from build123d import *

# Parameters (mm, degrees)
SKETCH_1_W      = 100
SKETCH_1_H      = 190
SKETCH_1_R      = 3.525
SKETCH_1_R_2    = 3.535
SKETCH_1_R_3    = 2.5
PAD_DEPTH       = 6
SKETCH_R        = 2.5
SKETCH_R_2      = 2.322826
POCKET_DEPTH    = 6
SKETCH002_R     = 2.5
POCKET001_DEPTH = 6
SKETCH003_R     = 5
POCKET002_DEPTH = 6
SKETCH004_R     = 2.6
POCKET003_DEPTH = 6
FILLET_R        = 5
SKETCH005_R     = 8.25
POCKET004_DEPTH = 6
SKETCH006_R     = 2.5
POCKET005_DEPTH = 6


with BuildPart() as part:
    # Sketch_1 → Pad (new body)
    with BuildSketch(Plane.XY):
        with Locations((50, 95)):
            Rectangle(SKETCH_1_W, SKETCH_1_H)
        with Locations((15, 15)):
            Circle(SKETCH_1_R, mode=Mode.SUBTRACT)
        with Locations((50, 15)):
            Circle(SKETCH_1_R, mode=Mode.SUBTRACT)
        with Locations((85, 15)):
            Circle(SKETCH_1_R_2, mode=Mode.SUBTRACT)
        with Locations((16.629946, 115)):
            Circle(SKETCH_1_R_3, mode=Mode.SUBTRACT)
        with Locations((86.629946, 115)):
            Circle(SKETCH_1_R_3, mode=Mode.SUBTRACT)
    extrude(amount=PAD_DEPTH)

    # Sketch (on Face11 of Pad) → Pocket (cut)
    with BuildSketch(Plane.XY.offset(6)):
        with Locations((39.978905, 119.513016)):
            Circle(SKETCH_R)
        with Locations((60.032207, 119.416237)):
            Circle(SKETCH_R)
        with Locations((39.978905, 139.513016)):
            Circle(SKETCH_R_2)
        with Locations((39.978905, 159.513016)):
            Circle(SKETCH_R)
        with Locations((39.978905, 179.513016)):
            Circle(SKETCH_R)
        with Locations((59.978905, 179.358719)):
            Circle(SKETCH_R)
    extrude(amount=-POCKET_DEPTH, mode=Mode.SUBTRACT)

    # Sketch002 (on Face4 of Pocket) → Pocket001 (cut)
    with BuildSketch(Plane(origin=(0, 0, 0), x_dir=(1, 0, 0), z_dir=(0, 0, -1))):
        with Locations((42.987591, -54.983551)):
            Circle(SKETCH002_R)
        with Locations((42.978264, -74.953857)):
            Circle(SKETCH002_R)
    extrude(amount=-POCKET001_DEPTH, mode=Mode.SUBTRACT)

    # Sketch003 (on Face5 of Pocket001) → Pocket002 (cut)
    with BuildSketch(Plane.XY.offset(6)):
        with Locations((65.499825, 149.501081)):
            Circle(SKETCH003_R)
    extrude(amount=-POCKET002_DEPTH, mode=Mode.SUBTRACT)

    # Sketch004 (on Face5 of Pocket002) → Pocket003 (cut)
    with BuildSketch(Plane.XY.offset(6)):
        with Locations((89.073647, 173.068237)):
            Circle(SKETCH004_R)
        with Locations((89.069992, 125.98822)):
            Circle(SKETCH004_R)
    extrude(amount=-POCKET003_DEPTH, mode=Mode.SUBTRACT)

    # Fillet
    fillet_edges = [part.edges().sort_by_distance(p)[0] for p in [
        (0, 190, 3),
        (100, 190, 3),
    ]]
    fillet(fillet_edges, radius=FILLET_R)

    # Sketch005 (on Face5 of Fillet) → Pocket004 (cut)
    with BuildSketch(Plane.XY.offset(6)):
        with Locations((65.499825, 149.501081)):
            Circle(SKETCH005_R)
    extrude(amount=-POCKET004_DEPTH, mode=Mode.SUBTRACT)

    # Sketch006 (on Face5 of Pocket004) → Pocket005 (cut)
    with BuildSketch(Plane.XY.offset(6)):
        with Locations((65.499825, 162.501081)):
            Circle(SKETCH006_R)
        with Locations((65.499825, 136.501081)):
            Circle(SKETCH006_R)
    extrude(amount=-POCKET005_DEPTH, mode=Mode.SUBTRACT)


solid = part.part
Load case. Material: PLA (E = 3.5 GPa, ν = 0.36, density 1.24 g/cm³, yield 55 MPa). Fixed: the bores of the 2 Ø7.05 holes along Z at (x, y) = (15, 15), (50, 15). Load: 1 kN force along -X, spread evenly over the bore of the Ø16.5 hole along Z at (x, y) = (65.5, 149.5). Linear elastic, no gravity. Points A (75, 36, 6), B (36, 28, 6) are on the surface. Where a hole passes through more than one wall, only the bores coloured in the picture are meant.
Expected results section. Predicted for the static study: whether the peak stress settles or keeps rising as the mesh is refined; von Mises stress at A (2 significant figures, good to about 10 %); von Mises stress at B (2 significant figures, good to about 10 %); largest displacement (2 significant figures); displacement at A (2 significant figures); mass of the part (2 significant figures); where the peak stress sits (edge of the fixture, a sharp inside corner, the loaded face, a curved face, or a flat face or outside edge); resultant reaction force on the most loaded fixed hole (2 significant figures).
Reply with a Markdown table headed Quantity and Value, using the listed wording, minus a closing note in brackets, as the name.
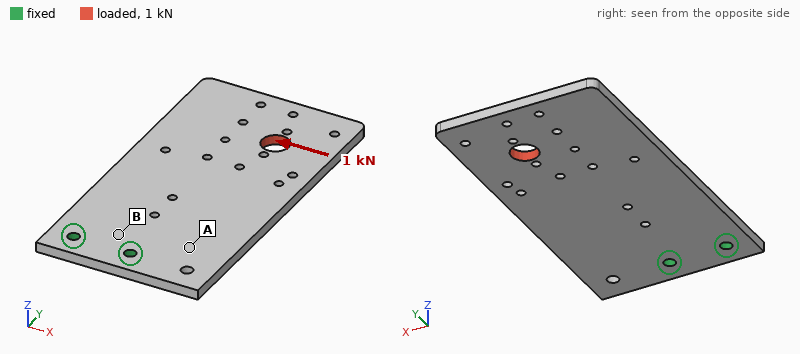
| Quantity | Value |
|---|---|
| whether the peak stress settles or keeps rising as the mesh is refined | keeps rising |
| von Mises stress at A | 6.9 MPa |
| von Mises stress at B | 14 MPa |
| largest displacement | 2.4 mm |
| displacement at A | 0.46 mm |
| mass of the part | 140 g |
| where the peak stress sits | edge of the fixture |
| resultant reaction force on the most loaded fixed hole | 3.4 kN |
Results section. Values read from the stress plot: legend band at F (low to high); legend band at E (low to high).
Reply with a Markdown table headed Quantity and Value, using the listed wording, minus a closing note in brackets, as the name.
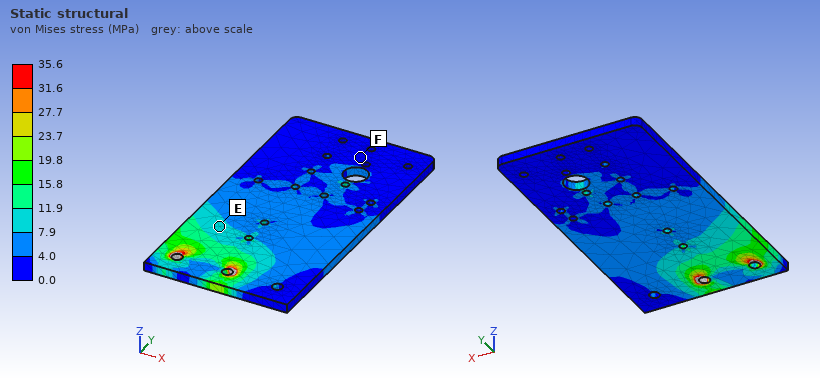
| Quantity | Value |
|---|---|
| legend band at F | 0.0 to 4.0 MPa |
| legend band at E | 7.9 to 11.9 MPa |
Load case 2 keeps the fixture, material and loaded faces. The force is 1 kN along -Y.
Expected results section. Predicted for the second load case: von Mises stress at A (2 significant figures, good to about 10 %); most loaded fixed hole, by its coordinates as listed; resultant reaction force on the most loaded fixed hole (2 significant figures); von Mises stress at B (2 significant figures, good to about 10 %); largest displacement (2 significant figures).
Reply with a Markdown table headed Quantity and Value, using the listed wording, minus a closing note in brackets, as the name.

| Quantity | Value |
|---|---|
| von Mises stress at A | 3.0 MPa |
| most loaded fixed hole, by its coordinates as listed | (50, 15) |
| resultant reaction force on the most loaded fixed hole | 1.3 kN |
| von Mises stress at B | 3.6 MPa |
| largest displacement | 0.56 mm |
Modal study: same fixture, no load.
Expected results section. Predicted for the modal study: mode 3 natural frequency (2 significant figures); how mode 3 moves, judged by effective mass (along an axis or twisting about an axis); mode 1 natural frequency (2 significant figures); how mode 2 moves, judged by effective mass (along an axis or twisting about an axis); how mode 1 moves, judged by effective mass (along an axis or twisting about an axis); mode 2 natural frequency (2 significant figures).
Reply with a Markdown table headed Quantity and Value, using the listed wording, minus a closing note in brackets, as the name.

| Quantity | Value |
|---|---|
| mode 3 natural frequency | 310 Hz |
| how mode 3 moves, judged by effective mass | along Z |
| mode 1 natural frequency | 53 Hz |
| how mode 2 moves, judged by effective mass | twisting about Y |
| how mode 1 moves, judged by effective mass | along Z |
| mode 2 natural frequency | 180 Hz |
